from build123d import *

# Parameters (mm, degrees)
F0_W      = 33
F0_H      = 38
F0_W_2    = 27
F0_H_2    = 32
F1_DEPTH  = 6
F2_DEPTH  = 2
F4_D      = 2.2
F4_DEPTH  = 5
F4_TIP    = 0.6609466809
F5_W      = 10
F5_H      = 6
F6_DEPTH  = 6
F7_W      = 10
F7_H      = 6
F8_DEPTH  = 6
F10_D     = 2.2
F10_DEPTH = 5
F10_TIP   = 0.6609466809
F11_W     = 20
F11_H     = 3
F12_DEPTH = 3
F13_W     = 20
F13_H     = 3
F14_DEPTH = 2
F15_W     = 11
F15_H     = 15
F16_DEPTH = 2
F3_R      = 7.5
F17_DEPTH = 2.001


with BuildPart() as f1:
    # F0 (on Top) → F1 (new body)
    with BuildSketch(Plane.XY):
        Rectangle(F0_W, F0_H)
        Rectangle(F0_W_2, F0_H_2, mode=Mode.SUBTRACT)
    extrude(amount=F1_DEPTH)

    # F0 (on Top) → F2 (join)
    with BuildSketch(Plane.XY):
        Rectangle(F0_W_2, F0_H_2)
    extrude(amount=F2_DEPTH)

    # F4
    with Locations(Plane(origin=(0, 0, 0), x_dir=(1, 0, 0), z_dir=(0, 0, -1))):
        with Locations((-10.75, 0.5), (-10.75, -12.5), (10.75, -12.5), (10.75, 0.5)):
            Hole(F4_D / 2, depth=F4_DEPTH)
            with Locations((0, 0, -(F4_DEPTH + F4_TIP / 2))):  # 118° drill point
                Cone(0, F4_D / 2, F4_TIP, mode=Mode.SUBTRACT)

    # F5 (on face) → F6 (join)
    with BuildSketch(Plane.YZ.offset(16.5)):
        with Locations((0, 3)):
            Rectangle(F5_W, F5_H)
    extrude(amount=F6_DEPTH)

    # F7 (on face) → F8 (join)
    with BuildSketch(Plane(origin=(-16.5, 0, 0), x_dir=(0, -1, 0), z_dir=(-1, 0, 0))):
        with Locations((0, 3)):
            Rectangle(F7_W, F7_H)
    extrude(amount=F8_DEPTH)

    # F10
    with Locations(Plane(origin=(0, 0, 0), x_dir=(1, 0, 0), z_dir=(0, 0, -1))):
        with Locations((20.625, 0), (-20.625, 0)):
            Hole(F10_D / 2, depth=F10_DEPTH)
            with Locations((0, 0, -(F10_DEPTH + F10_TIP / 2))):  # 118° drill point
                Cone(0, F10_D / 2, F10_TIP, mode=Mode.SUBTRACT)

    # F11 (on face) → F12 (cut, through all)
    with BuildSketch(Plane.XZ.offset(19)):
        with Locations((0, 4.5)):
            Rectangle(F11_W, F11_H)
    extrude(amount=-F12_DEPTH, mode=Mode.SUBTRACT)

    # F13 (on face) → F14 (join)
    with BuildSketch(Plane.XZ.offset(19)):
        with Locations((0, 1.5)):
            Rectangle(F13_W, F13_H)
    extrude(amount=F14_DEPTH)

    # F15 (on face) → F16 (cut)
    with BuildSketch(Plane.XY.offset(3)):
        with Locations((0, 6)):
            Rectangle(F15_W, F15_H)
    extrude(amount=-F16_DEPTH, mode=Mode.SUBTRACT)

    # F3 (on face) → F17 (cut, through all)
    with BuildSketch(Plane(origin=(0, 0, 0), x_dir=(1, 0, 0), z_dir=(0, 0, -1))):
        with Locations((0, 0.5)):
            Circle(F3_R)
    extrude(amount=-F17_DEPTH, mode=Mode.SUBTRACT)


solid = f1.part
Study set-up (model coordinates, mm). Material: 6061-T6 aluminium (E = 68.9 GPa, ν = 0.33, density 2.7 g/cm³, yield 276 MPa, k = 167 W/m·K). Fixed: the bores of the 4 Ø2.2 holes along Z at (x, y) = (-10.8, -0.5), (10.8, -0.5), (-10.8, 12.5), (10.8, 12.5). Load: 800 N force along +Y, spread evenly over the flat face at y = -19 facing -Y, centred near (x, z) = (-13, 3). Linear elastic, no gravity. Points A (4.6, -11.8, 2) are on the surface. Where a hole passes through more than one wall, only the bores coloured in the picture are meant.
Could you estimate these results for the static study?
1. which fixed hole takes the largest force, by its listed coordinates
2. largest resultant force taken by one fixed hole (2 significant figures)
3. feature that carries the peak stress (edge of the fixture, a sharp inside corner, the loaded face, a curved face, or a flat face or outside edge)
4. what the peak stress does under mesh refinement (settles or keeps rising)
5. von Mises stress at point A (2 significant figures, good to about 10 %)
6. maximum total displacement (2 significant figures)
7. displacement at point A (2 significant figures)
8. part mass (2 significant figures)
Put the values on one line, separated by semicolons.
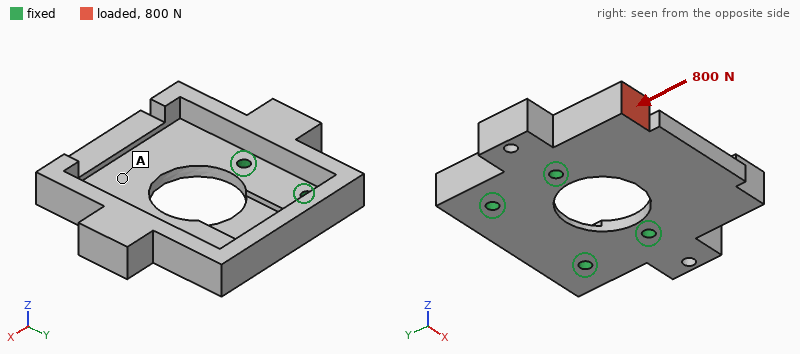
(-10.8, -0.5); 570 N; edge of the fixture; keeps rising; 8.0 MPa; 39 µm; 6.3 µm; 11 g
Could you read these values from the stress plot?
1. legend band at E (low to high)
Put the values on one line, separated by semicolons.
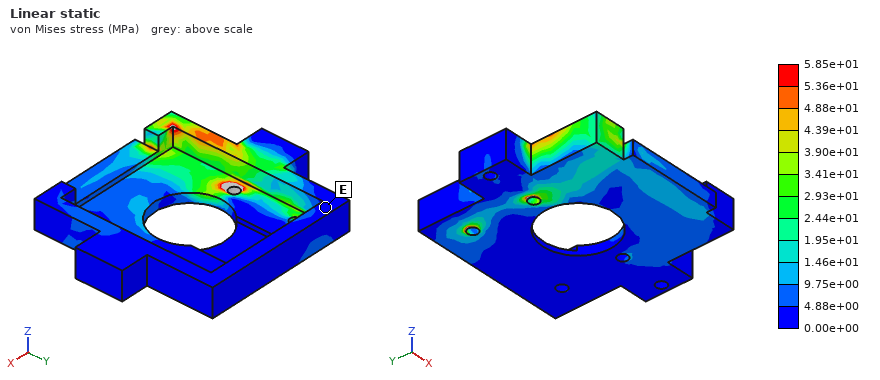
0.00e+00 to 4.88e+00 MPa
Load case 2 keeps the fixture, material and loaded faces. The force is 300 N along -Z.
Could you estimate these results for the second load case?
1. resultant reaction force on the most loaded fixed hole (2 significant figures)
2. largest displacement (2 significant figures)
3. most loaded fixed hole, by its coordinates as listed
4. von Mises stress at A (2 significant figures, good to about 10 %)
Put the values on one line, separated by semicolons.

680 N; 0.18 mm; (-10.8, -0.5); 39 MPa
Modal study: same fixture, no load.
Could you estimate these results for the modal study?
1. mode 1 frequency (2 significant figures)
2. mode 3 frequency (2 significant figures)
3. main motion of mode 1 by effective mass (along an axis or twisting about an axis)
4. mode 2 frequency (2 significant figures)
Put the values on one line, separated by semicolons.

6000 Hz; 9900 Hz; along Z; 8100 Hz
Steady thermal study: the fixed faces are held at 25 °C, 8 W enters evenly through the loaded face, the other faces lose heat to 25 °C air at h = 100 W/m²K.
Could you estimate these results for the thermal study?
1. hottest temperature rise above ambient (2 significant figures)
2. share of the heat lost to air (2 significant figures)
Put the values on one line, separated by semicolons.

21 K; 17 %
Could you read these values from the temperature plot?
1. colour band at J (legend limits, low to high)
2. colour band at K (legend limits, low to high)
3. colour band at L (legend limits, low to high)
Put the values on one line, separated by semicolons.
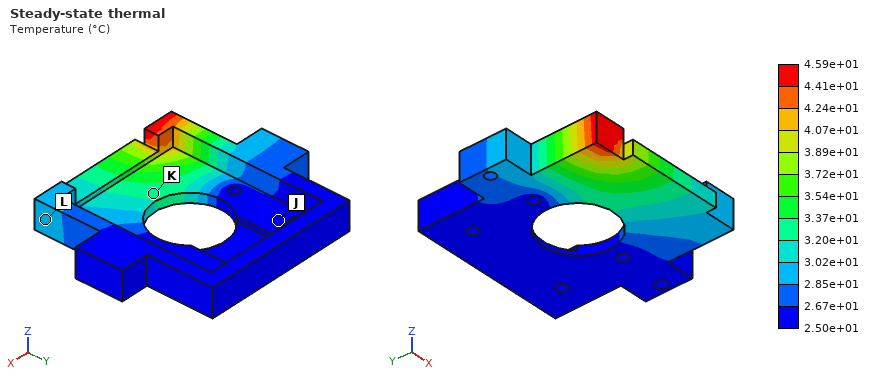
2.50e+01 to 2.67e+01 °C; 3.20e+01 to 3.37e+01 °C; 2.85e+01 to 3.02e+01 °C
